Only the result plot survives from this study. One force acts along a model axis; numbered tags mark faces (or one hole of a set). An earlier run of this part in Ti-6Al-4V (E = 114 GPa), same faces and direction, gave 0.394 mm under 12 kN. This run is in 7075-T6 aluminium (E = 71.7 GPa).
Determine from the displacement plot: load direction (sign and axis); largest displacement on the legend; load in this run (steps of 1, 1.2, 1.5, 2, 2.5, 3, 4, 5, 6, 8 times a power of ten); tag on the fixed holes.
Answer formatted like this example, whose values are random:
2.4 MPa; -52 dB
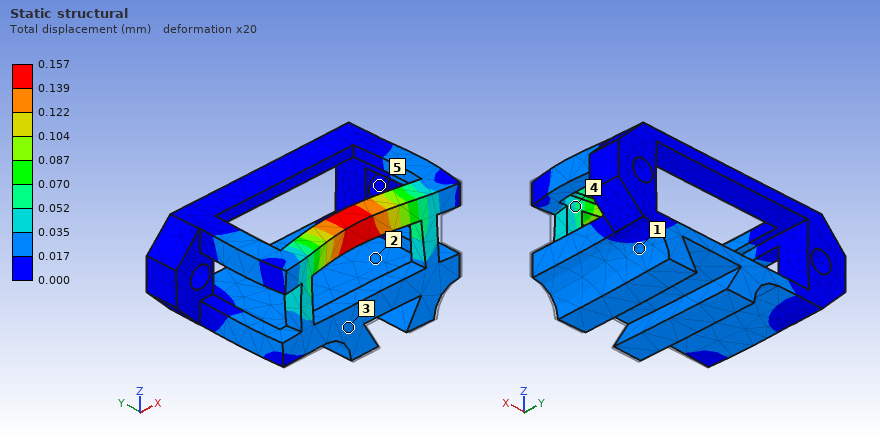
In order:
+Y; 0.157 mm; 3 kN; 5
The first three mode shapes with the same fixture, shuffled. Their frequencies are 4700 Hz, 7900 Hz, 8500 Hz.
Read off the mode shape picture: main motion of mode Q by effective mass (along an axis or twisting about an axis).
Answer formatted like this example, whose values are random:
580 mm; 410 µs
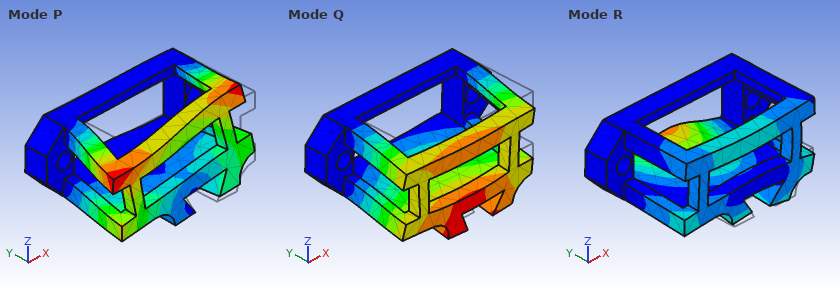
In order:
along Z
